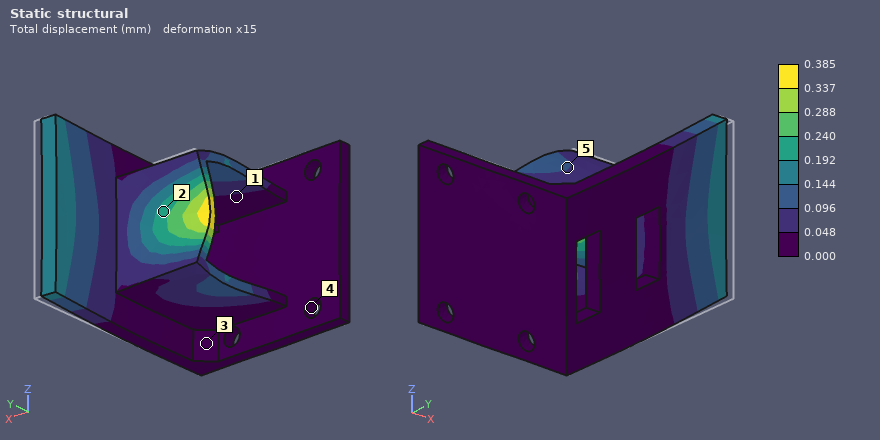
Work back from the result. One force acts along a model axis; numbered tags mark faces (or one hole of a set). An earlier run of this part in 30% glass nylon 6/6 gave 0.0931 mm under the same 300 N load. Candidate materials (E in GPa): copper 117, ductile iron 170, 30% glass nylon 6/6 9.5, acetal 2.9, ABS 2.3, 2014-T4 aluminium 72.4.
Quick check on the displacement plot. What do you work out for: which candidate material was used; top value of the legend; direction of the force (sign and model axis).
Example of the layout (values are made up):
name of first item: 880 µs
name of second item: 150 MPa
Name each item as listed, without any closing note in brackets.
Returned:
which candidate material was used: ABS
top value of the legend: 0.385 mm
direction of the force: -Y
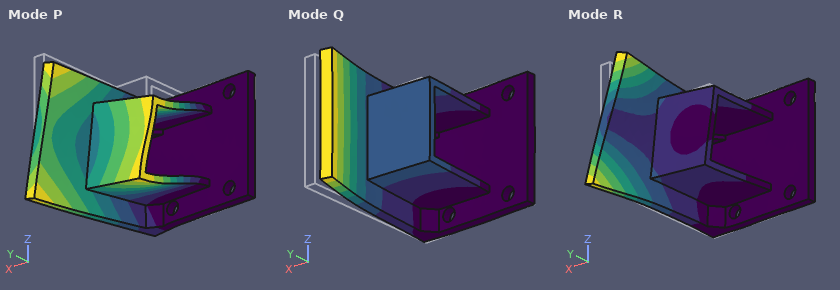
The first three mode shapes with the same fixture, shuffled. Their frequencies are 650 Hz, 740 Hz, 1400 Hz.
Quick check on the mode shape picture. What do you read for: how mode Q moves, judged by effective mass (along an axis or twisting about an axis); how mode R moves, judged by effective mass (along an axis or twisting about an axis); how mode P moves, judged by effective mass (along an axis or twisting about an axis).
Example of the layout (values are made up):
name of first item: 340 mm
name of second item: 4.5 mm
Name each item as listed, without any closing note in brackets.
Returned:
how mode Q moves, judged by effective mass: along X
how mode R moves, judged by effective mass: along Z
how mode P moves, judged by effective mass: along Z
